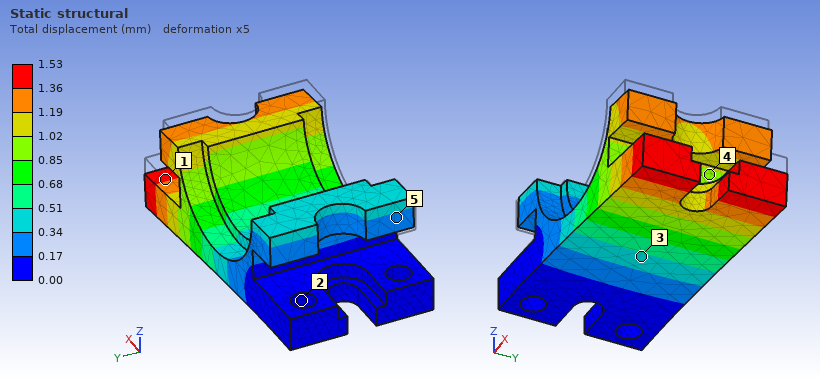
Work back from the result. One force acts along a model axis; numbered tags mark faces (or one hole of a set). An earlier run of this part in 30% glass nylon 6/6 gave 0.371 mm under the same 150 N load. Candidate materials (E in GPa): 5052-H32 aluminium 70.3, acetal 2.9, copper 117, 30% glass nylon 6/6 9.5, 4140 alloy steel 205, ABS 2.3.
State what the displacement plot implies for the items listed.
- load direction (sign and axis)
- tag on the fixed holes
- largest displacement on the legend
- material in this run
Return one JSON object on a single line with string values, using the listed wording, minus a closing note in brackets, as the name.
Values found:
{"load direction": "-Z", "tag on the fixed holes": "2", "largest displacement on the legend": "1.53 mm", "material in this run": "ABS"}
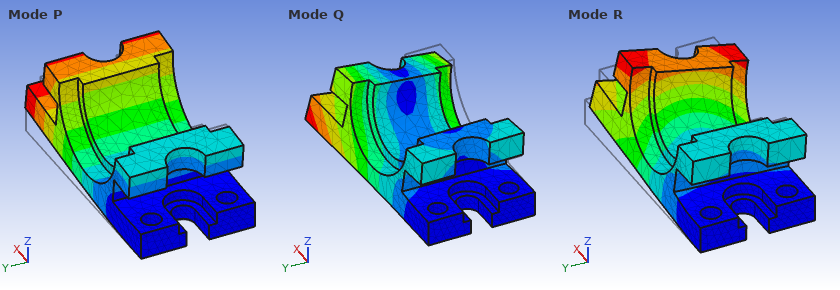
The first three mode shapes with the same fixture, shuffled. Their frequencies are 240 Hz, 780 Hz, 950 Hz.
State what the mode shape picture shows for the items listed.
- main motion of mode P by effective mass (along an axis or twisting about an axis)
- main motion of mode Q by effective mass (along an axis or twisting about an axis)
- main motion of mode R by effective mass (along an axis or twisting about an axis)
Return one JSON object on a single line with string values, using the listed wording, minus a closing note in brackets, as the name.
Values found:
{"main motion of mode P by effective mass": "along Z", "main motion of mode Q by effective mass": "along Y", "main motion of mode R by effective mass": "along Y"}
